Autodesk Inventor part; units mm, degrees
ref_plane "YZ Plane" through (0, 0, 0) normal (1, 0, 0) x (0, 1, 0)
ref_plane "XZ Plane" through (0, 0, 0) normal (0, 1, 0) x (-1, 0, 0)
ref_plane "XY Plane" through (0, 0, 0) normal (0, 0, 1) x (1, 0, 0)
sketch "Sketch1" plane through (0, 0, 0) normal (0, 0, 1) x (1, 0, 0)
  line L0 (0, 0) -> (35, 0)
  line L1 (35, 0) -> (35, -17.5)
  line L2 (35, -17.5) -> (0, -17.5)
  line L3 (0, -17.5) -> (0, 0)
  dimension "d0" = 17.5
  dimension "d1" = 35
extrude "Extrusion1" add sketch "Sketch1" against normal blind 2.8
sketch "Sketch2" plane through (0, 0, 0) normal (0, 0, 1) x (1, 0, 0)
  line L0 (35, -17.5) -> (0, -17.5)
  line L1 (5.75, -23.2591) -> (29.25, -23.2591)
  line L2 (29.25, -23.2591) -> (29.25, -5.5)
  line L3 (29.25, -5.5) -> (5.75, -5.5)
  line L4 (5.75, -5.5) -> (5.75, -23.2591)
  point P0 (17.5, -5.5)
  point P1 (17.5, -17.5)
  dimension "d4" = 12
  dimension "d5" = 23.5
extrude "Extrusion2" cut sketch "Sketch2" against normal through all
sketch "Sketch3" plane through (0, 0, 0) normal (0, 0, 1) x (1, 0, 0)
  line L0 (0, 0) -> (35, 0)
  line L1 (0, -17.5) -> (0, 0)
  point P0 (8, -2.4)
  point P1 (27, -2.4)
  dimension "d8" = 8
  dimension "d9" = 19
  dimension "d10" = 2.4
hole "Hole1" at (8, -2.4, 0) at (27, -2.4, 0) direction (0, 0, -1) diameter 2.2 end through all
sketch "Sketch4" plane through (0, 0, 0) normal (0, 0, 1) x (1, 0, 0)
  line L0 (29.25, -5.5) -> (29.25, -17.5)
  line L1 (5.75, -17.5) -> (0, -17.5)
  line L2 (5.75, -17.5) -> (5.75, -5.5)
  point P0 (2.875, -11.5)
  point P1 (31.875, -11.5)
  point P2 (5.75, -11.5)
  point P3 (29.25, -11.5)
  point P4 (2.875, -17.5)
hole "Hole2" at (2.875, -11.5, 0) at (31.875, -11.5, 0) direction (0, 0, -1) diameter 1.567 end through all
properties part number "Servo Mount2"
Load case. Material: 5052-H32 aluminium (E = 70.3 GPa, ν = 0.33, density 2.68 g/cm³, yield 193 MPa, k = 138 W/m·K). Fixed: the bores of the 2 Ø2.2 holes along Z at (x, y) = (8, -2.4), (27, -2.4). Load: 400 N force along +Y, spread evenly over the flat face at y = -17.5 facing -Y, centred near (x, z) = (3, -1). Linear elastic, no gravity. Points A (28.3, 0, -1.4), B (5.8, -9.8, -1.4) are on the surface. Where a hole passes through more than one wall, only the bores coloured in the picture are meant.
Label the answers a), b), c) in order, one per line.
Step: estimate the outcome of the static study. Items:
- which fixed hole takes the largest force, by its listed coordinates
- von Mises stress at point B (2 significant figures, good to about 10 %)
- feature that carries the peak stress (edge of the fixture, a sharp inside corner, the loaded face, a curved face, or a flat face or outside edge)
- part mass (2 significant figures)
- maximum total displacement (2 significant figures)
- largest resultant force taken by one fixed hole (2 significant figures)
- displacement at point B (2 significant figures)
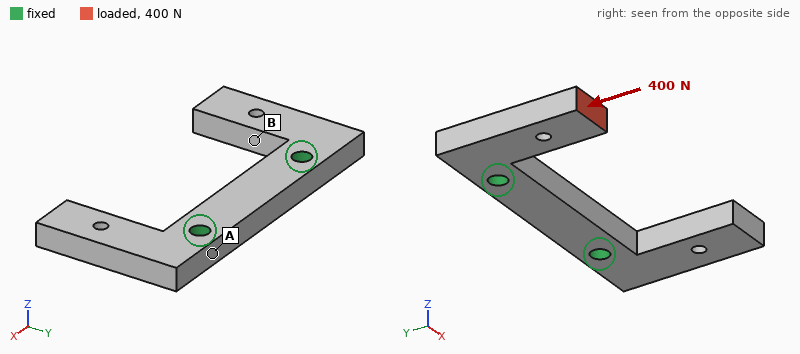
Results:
a) (8, -2.4)
b) 30 MPa
c) edge of the fixture
d) 2.4 g
e) 55 µm
f) 430 N
g) 23 µm
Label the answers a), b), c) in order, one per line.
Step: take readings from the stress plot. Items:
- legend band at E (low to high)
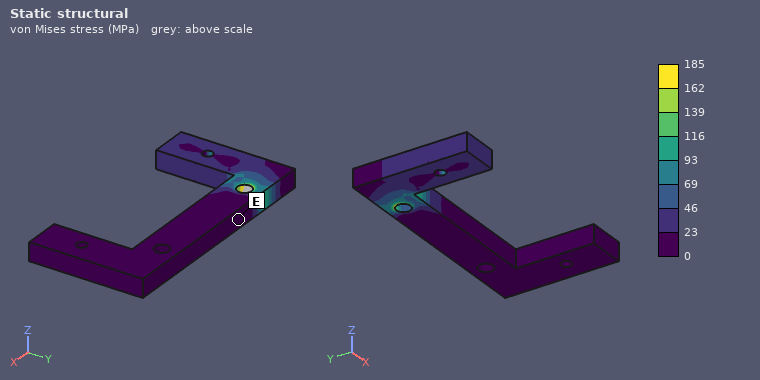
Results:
a) 0 to 23 MPa
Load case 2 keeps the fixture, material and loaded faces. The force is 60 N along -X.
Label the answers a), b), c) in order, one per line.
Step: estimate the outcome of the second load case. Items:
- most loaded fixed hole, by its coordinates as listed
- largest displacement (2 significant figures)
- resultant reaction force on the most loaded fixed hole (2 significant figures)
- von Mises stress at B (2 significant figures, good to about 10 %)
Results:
a) (8, -2.4)
b) 48 µm
c) 47 N
d) 32 MPa
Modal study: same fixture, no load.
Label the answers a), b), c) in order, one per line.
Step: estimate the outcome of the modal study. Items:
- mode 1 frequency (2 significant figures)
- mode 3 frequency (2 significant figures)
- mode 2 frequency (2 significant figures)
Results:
a) 8100 Hz
b) 13 kHz
c) 8100 Hz
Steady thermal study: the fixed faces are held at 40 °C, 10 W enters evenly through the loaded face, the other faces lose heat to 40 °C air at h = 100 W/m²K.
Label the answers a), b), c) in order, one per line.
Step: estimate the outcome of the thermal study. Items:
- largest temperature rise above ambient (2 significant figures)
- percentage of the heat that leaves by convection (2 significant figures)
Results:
a) 74 K
b) 12 %
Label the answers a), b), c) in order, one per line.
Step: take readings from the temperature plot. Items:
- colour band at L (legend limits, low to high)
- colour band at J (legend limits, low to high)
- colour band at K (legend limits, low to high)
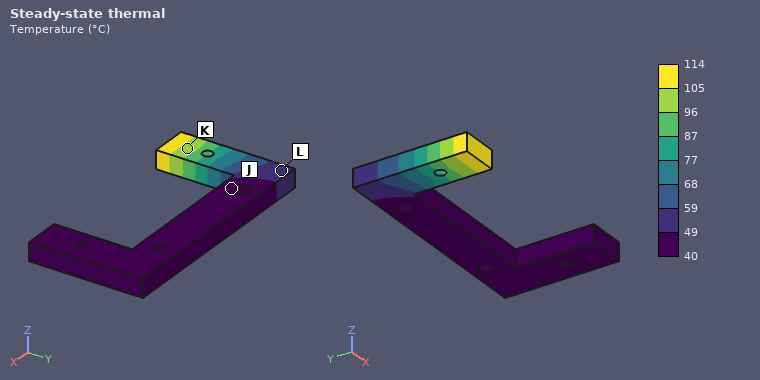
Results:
a) 49 to 59 °C
b) 40 to 49 °C
c) 96 to 105 °C
